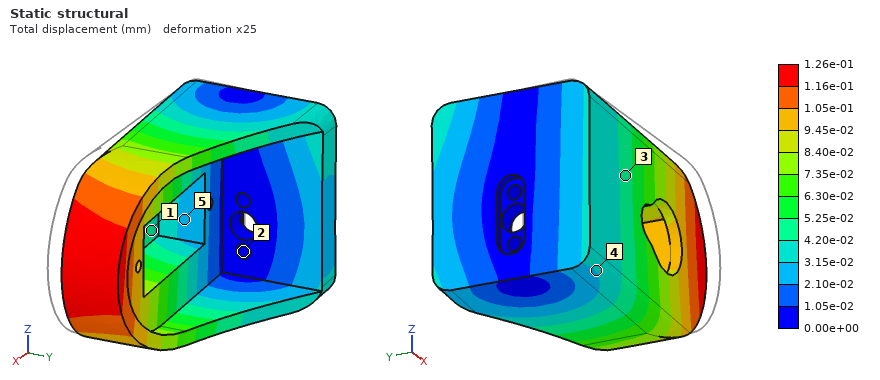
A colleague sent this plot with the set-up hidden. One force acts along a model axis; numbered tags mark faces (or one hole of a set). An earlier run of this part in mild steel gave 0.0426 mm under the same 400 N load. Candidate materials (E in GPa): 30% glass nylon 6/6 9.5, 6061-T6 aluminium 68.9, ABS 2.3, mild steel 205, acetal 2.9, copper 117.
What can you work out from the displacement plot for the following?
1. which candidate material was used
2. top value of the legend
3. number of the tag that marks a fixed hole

6061-T6 aluminium
1.26e-01 mm
2
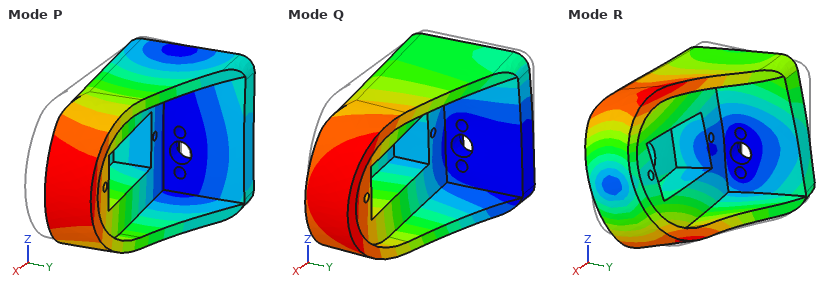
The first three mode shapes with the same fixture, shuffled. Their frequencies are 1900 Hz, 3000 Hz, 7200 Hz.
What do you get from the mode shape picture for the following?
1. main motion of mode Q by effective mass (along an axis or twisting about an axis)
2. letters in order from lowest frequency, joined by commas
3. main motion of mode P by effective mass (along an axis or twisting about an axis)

along Z
P, Q, R
along Y
